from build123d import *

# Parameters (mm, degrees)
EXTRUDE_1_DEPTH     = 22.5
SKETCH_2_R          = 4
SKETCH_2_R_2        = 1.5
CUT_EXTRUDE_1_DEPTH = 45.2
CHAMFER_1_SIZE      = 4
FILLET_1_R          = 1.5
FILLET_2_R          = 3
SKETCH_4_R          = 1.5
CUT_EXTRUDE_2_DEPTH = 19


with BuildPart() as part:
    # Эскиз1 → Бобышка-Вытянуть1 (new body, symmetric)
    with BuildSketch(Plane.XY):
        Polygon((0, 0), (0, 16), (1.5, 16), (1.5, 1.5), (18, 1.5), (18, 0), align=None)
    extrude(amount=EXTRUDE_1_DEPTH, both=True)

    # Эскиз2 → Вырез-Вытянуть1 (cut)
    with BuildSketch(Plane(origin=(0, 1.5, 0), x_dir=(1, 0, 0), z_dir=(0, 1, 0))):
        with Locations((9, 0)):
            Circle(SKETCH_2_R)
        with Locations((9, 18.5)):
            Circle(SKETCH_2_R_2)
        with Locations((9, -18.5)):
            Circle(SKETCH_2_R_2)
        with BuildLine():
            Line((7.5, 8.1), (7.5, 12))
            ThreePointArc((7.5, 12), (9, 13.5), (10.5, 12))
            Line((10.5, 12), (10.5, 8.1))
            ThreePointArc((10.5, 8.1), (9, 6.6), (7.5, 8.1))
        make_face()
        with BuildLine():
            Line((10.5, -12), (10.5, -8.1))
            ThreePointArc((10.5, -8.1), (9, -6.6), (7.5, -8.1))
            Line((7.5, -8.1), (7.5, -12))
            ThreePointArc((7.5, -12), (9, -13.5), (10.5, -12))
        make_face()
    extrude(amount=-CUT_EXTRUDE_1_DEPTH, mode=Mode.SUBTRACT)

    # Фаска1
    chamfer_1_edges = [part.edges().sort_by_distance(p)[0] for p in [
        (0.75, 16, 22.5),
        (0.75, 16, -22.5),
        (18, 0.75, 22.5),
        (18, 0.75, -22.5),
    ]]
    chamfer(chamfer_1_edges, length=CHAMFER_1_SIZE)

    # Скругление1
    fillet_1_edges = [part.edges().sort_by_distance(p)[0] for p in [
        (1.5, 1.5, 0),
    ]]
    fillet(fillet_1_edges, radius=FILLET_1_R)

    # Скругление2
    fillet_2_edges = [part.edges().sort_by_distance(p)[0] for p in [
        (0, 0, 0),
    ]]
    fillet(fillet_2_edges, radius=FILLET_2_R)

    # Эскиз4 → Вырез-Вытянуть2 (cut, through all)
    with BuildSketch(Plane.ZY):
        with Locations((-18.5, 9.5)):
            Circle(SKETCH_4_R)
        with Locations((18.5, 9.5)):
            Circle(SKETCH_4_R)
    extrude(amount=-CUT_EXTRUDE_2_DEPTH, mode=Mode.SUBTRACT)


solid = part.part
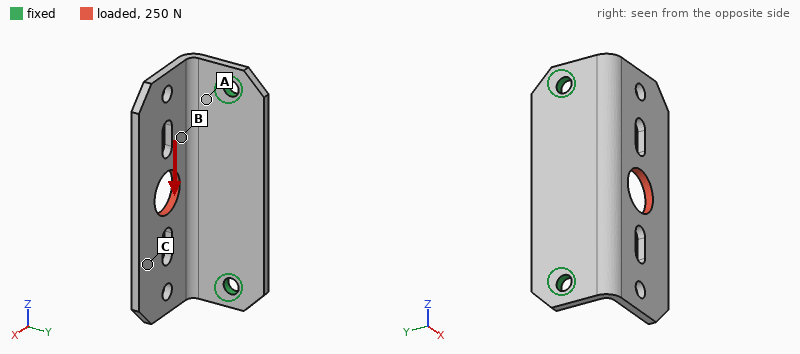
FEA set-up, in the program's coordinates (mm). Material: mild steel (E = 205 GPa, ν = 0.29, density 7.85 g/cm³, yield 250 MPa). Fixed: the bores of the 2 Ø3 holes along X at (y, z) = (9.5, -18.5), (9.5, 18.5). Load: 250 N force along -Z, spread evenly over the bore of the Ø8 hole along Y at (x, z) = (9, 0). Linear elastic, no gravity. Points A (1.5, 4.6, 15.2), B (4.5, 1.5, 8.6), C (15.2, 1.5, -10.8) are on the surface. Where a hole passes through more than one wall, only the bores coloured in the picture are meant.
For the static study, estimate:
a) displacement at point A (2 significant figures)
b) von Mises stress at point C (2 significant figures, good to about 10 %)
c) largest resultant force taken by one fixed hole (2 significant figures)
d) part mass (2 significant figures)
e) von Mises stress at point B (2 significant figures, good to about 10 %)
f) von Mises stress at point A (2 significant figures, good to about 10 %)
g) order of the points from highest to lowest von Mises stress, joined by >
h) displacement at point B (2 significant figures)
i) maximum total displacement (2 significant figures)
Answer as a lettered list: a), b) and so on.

a) 3.4 µm
b) 8.9 MPa
c) 150 N
d) 15 g
e) 23 MPa
f) 36 MPa
g) A > B > C
h) 5.4 µm
i) 22 µm
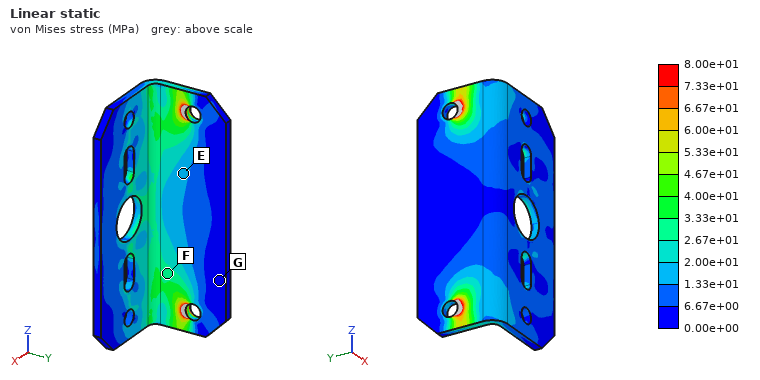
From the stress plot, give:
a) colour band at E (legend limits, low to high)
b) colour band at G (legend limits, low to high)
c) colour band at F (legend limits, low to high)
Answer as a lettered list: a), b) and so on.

a) 1.33e+01 to 2.00e+01 MPa
b) 0.00e+00 to 6.67e+00 MPa
c) 2.67e+01 to 3.33e+01 MPa
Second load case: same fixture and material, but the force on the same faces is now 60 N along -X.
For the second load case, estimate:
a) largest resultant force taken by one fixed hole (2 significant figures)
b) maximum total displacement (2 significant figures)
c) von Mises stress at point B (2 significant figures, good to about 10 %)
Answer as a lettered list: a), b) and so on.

a) 31 N
b) 22 µm
c) 5.6 MPa
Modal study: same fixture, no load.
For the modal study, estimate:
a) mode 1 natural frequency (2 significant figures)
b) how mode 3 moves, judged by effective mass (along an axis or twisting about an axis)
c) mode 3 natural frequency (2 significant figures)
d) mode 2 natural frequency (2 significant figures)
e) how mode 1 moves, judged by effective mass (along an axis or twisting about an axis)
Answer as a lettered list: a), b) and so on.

a) 2300 Hz
b) along X
c) 6400 Hz
d) 4000 Hz
e) along Y
